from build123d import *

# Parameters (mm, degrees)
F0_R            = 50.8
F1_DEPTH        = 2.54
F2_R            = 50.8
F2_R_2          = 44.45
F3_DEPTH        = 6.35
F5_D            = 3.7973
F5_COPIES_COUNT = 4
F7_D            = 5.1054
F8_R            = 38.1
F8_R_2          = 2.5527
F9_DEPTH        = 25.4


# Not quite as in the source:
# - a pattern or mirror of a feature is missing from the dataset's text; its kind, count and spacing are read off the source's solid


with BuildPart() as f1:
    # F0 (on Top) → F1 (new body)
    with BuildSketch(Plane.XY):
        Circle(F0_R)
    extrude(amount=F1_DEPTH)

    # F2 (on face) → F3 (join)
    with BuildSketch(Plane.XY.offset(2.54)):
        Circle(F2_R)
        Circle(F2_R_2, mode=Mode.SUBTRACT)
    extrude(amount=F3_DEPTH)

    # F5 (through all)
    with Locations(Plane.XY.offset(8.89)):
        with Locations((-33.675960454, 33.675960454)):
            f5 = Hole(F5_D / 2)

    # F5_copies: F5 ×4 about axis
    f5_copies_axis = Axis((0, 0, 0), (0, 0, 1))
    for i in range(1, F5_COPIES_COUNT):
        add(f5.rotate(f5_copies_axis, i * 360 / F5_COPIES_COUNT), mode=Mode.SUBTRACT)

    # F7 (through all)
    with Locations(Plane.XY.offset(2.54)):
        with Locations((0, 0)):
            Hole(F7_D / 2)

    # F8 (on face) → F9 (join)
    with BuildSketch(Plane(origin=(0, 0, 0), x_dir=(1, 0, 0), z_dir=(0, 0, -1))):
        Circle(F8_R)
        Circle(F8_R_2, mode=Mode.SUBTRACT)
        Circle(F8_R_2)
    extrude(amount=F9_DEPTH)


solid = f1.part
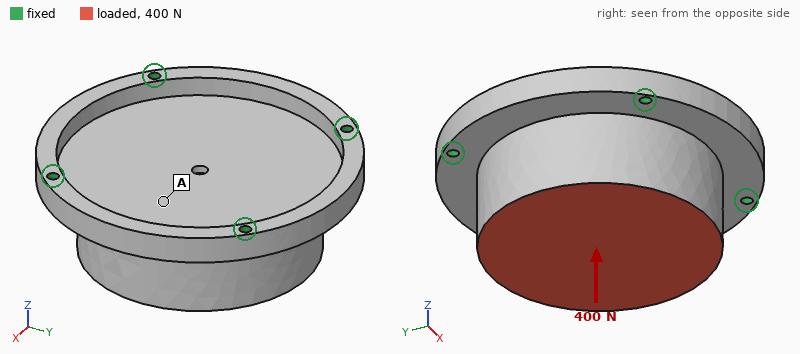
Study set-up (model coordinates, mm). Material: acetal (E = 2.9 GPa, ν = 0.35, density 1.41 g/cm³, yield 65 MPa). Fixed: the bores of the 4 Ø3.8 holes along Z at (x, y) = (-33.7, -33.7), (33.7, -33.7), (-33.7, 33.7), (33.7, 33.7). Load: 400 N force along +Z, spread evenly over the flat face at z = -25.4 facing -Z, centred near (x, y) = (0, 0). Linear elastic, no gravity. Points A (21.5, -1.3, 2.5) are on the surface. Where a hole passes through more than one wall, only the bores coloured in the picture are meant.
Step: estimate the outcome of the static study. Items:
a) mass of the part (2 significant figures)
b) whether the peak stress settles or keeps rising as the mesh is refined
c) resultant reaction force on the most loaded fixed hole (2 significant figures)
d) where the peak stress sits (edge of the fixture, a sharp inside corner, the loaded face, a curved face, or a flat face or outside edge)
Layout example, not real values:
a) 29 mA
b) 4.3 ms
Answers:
a) 210 g
b) keeps rising
c) 120 N
d) edge of the fixture
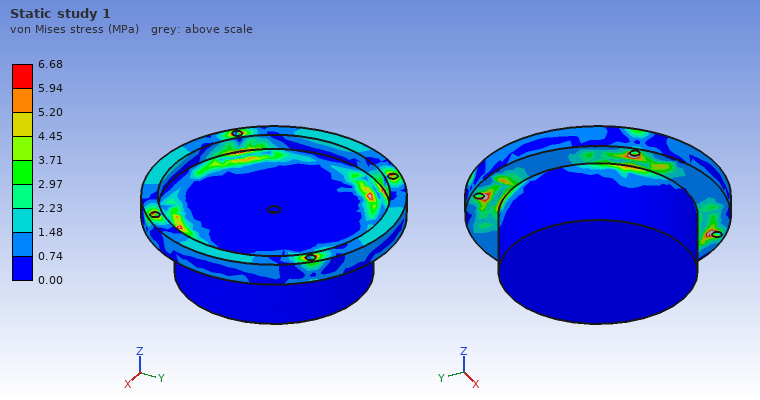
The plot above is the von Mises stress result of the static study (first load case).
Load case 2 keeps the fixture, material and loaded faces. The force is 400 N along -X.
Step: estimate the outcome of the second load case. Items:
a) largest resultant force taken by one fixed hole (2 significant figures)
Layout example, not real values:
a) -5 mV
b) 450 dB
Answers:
a) 140 N
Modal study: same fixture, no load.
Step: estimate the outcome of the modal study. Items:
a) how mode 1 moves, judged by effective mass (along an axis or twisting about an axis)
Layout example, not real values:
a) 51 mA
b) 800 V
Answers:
a) along Z
